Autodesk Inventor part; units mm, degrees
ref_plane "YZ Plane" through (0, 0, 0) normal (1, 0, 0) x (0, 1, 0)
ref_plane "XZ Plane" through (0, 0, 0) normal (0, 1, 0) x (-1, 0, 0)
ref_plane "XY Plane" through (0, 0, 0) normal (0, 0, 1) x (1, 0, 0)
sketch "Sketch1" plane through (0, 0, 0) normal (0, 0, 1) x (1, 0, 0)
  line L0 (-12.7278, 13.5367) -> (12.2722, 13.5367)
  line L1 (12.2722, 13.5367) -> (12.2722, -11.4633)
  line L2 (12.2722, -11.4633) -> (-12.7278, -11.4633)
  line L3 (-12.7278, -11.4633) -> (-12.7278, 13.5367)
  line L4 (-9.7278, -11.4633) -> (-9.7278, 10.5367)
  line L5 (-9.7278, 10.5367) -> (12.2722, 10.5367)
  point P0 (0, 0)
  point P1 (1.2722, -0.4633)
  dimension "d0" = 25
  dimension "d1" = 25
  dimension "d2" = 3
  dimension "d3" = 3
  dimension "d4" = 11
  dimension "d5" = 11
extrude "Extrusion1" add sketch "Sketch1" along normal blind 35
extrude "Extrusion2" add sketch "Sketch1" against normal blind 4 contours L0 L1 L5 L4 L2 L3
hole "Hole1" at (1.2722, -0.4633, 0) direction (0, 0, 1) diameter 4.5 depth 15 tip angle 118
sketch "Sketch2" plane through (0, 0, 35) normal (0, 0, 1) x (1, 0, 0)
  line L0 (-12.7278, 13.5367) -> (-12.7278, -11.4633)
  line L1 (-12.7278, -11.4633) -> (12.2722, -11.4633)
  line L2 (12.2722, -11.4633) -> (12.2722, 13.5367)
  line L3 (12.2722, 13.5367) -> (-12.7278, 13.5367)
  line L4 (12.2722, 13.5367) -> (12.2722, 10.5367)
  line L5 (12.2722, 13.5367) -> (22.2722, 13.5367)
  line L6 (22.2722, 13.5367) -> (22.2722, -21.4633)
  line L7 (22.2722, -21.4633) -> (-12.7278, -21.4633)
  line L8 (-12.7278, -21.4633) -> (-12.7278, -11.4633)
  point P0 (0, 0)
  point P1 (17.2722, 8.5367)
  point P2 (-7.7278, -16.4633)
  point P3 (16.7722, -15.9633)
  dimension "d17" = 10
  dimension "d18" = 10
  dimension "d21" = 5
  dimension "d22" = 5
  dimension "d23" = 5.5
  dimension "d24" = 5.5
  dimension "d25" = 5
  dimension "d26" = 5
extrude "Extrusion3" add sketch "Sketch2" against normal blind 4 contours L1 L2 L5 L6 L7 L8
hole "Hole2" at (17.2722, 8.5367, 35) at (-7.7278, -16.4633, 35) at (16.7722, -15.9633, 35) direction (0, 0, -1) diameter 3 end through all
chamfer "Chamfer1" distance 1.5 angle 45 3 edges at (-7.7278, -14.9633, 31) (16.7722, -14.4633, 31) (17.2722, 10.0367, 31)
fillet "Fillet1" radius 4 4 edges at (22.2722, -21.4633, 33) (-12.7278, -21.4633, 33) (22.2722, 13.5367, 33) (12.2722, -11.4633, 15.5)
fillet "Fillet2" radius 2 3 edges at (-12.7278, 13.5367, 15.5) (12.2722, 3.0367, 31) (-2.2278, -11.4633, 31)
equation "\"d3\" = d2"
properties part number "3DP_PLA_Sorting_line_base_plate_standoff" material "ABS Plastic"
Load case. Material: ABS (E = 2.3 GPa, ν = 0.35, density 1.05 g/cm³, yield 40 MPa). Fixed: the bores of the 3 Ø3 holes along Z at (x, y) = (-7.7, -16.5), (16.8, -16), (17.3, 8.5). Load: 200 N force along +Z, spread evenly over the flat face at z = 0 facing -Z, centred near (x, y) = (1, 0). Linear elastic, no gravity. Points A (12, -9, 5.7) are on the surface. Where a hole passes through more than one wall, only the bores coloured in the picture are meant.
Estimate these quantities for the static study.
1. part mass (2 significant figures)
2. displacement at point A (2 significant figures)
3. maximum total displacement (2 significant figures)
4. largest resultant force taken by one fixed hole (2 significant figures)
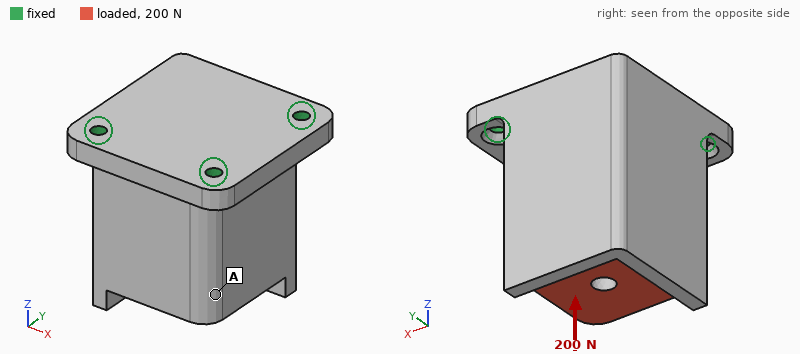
26 g
0.15 mm
0.27 mm
130 N
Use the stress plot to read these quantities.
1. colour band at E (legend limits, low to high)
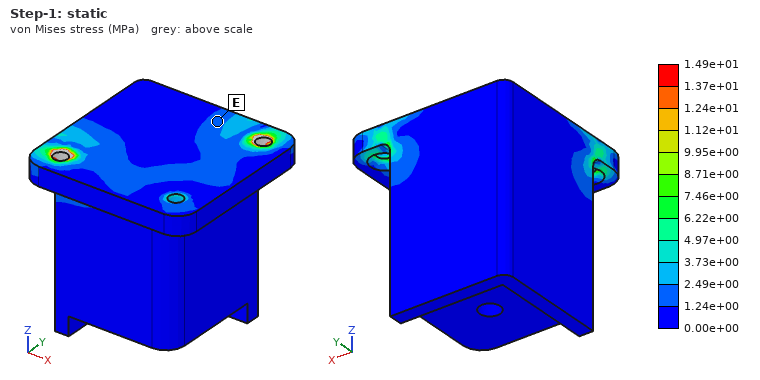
1.24e+00 to 2.49e+00 MPa
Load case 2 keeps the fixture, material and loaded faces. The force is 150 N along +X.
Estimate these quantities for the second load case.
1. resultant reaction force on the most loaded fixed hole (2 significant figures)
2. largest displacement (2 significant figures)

240 N
0.69 mm
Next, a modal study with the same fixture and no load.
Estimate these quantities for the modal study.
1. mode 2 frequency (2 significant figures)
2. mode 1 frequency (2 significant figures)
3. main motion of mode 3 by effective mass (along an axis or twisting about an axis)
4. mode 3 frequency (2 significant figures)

1800 Hz
710 Hz
along Z
2700 Hz
